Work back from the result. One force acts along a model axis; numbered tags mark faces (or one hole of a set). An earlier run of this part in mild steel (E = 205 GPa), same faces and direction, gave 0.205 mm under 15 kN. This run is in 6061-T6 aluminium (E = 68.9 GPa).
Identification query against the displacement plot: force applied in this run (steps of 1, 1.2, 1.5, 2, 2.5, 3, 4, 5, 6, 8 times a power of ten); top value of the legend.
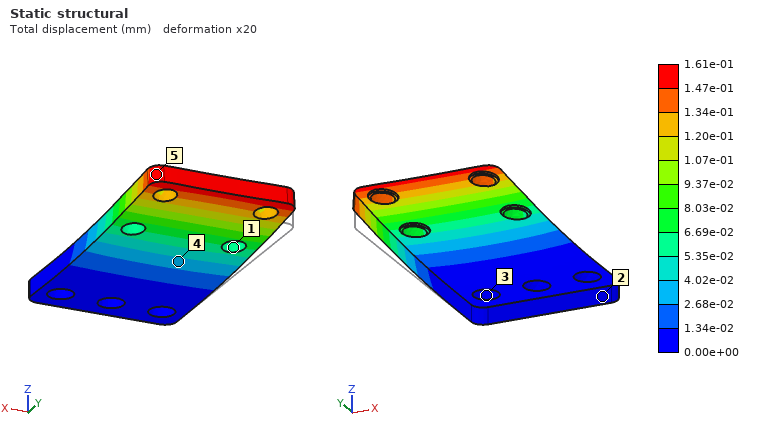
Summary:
4 kN
1.61e-01 mm
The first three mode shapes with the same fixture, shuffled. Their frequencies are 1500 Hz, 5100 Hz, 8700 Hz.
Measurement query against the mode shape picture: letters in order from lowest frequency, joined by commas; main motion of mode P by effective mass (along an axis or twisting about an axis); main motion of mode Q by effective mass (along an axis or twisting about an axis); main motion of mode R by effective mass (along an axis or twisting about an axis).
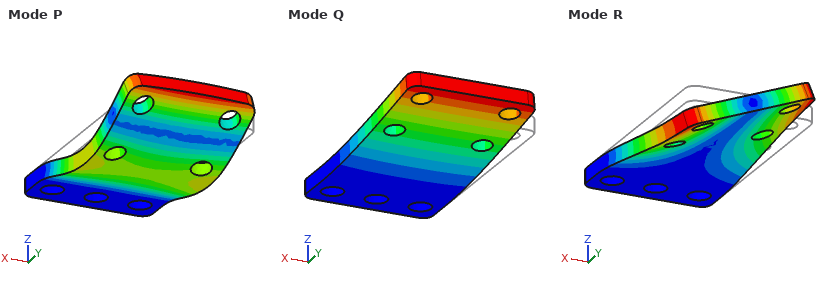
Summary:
Q, R, P
along Z
along Z
twisting about Y
